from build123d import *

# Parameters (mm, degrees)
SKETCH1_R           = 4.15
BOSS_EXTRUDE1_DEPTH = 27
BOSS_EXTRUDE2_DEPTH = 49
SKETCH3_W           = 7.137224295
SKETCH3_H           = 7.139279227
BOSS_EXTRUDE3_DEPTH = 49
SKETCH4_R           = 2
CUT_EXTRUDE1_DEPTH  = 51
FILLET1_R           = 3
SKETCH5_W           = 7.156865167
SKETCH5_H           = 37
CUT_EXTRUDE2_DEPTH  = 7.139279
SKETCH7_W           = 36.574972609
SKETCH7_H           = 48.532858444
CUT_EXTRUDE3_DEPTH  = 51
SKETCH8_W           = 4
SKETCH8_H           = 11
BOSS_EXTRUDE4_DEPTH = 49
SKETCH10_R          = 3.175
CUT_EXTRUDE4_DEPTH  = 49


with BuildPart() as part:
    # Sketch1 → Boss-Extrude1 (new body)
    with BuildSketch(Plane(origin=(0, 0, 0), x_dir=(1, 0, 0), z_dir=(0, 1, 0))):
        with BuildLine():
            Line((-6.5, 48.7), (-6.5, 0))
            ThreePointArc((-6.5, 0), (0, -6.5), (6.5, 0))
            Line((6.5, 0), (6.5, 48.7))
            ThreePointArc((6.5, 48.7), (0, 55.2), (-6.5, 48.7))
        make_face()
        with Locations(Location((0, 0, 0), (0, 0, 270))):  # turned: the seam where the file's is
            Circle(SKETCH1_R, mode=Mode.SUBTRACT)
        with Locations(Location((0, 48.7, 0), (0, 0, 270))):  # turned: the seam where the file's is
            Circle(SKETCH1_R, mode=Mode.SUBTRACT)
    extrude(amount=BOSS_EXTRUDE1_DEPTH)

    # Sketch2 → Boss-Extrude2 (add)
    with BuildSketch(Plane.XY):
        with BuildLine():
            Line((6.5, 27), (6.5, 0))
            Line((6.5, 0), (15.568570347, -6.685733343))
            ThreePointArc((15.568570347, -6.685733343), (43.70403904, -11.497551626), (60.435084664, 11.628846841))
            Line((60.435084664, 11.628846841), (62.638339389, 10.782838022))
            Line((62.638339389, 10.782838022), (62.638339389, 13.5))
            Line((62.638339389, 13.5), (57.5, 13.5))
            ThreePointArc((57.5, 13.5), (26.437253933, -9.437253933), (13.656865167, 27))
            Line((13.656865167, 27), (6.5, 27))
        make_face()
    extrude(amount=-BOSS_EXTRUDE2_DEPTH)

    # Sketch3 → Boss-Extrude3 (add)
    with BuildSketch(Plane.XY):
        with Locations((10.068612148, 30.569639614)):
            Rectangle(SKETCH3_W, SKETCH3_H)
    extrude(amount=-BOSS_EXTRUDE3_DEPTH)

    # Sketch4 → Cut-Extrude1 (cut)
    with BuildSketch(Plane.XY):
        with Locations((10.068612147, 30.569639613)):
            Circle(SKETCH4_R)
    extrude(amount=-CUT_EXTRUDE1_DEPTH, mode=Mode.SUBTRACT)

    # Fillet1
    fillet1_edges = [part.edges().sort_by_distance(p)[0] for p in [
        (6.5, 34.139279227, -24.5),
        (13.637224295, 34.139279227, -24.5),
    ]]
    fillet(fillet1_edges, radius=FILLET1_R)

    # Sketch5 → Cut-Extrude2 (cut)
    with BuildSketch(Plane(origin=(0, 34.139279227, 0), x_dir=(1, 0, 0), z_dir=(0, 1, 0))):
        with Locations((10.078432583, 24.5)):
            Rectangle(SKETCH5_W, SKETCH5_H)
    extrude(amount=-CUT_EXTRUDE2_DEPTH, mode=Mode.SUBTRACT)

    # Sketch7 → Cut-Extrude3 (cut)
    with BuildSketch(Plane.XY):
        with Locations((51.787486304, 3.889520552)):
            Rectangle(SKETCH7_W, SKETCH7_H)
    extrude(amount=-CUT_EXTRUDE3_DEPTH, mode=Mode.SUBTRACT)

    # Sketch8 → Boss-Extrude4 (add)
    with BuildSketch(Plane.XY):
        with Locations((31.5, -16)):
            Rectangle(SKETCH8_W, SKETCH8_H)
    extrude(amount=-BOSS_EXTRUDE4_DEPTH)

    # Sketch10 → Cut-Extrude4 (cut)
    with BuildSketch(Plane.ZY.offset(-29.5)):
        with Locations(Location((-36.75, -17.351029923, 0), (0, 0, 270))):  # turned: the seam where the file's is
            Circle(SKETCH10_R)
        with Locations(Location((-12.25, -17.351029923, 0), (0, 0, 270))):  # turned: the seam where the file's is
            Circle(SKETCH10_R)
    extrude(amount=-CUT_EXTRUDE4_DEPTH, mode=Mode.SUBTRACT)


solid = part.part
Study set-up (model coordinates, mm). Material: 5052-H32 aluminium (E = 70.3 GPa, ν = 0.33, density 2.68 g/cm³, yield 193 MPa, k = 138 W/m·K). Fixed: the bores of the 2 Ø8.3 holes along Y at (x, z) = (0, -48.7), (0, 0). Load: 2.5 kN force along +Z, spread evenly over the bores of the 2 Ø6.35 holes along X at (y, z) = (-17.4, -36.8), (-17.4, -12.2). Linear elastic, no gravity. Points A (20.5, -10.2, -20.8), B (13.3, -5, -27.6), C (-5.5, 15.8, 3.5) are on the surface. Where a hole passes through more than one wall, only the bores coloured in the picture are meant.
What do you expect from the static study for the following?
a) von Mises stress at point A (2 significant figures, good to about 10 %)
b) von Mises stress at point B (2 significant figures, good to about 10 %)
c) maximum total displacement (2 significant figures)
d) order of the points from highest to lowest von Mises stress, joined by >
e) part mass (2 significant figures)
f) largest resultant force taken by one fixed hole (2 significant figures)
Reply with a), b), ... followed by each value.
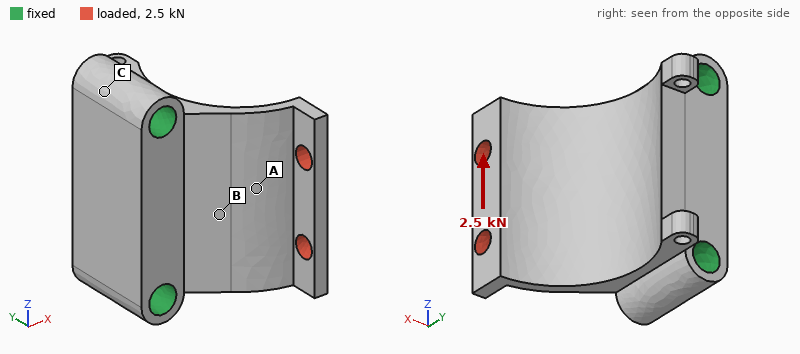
a) 72 MPa
b) 37 MPa
c) 0.15 mm
d) A > B > C
e) 79 g
f) 2.5 kN
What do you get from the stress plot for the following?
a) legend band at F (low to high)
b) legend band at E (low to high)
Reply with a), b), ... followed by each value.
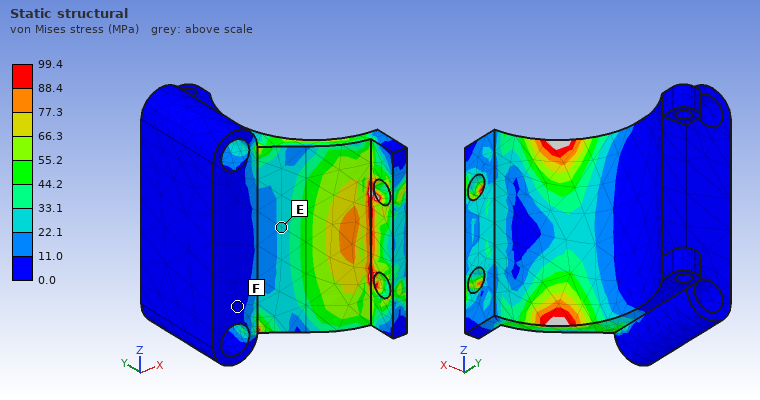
a) 0.0 to 11.0 MPa
b) 22.1 to 33.1 MPa
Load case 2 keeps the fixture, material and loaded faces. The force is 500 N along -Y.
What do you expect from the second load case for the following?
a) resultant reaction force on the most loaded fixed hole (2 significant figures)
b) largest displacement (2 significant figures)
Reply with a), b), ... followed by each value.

a) 250 N
b) 0.30 mm
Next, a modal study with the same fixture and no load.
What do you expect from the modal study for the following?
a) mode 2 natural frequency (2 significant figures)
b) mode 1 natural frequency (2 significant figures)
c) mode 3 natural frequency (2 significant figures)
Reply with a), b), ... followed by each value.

a) 4500 Hz
b) 2600 Hz
c) 14 kHz
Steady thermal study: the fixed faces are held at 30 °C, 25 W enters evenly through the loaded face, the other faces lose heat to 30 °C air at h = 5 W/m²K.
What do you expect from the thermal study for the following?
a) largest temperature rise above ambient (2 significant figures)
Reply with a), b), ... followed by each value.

a) 45 K
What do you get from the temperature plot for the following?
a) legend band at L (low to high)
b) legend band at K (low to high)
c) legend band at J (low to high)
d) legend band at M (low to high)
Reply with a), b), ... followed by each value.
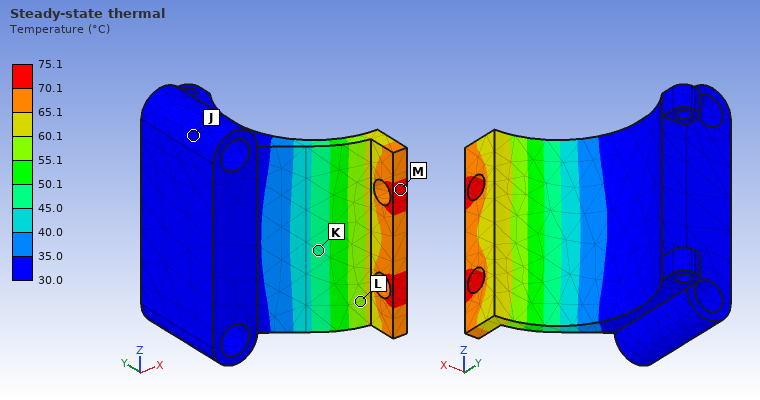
a) 55.1 to 60.1 °C
b) 45.0 to 50.1 °C
c) 30.0 to 35.0 °C
d) 70.1 to 75.1 °C
